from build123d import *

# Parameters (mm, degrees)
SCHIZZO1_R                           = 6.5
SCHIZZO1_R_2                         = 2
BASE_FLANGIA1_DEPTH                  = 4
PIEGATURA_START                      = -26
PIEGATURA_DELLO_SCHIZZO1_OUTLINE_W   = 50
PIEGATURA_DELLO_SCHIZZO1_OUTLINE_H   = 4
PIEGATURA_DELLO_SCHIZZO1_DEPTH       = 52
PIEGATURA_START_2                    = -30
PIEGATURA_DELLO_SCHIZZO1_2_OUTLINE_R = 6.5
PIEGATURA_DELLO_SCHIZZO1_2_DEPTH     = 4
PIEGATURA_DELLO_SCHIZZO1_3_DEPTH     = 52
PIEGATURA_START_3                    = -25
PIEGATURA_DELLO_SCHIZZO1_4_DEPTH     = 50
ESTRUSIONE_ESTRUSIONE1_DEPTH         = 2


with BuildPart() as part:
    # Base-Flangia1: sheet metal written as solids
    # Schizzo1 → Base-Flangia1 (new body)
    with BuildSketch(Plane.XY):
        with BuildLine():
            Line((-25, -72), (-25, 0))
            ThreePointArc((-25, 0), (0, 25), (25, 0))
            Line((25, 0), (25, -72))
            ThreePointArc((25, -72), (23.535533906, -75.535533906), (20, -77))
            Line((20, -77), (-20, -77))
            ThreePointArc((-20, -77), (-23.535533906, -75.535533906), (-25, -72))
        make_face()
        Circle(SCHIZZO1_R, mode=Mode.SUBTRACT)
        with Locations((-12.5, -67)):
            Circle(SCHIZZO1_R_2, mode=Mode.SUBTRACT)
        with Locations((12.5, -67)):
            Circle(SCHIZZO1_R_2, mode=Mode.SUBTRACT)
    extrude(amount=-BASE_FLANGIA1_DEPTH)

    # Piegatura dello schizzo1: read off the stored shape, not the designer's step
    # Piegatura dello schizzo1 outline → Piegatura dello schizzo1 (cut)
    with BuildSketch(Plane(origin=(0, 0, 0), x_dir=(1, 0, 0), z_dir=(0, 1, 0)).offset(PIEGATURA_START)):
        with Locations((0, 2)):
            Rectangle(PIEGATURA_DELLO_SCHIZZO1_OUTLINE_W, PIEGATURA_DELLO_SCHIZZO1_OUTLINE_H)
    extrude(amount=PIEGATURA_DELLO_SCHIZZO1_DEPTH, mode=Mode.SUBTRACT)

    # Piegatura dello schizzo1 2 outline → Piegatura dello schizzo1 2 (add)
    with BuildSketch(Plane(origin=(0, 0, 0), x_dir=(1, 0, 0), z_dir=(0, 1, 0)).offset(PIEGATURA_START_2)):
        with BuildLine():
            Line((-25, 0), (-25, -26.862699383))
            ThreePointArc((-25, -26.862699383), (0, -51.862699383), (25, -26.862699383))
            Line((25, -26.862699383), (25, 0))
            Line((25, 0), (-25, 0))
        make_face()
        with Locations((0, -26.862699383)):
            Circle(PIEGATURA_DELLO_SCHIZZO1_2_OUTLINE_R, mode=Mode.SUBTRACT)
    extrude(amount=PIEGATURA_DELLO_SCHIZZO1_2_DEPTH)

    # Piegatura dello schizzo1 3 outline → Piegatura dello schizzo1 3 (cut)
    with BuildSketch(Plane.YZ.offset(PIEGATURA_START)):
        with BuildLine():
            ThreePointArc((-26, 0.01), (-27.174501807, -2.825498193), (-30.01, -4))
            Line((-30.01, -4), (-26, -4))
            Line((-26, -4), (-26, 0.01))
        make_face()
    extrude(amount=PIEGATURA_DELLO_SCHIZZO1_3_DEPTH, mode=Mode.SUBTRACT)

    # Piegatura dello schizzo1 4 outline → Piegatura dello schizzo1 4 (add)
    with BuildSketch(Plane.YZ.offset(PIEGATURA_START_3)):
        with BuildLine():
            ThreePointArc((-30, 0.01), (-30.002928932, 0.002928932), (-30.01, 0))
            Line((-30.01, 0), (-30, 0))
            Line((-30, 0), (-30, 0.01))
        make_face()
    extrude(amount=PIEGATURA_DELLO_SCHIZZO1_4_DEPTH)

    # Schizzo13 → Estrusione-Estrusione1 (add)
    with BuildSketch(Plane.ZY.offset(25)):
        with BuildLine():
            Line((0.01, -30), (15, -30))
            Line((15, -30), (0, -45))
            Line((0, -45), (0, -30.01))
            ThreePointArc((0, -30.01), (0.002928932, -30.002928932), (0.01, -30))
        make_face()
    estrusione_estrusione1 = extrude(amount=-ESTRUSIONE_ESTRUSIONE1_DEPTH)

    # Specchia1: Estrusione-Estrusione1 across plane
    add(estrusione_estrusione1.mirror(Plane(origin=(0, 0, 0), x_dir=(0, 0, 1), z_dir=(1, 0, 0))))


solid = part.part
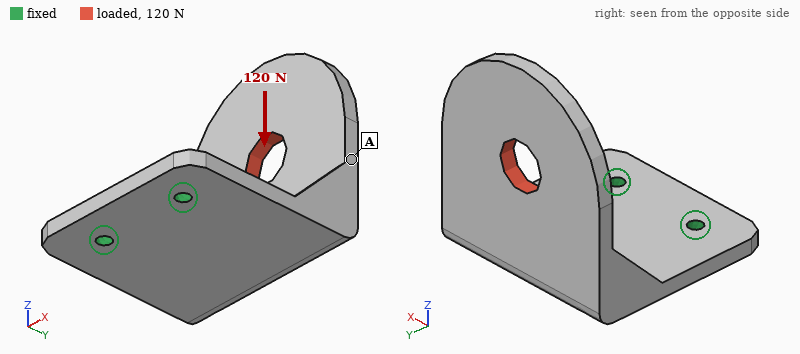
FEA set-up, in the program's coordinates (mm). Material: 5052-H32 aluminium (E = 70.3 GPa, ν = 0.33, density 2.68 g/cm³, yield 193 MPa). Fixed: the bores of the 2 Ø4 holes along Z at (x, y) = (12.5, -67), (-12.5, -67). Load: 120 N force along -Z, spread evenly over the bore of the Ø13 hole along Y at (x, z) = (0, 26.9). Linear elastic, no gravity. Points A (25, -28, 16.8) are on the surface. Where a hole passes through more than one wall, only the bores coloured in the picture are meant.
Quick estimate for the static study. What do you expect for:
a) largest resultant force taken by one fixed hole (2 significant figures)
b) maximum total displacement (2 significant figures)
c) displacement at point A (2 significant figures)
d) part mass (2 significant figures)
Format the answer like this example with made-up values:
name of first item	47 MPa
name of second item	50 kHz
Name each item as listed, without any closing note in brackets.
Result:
largest resultant force taken by one fixed hole	60 N
maximum total displacement	0.28 mm
displacement at point A	0.15 mm
part mass	51 g
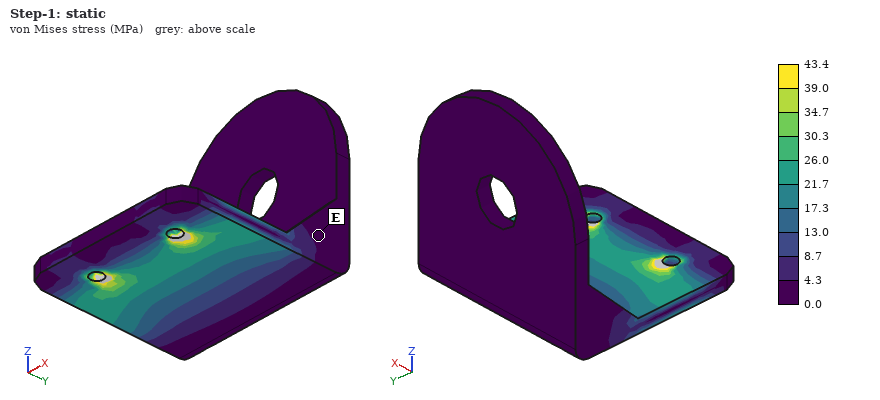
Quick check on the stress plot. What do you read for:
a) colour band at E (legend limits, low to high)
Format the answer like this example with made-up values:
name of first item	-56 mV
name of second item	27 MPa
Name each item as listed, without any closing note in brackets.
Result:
colour band at E	0.0 to 4.3 MPa
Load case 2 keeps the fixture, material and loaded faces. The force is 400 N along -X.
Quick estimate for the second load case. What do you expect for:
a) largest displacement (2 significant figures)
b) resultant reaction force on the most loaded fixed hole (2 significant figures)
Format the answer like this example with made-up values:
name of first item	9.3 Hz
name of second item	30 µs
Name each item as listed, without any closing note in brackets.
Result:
largest displacement	0.47 mm
resultant reaction force on the most loaded fixed hole	690 N
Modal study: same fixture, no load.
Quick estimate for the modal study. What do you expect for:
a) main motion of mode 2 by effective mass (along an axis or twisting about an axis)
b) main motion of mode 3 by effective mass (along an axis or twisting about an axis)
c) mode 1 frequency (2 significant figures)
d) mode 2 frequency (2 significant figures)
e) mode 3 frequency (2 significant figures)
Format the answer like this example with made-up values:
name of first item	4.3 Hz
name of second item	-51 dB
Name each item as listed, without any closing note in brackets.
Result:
main motion of mode 2 by effective mass	along X
main motion of mode 3 by effective mass	along Z
mode 1 frequency	620 Hz
mode 2 frequency	1100 Hz
mode 3 frequency	1900 Hz
